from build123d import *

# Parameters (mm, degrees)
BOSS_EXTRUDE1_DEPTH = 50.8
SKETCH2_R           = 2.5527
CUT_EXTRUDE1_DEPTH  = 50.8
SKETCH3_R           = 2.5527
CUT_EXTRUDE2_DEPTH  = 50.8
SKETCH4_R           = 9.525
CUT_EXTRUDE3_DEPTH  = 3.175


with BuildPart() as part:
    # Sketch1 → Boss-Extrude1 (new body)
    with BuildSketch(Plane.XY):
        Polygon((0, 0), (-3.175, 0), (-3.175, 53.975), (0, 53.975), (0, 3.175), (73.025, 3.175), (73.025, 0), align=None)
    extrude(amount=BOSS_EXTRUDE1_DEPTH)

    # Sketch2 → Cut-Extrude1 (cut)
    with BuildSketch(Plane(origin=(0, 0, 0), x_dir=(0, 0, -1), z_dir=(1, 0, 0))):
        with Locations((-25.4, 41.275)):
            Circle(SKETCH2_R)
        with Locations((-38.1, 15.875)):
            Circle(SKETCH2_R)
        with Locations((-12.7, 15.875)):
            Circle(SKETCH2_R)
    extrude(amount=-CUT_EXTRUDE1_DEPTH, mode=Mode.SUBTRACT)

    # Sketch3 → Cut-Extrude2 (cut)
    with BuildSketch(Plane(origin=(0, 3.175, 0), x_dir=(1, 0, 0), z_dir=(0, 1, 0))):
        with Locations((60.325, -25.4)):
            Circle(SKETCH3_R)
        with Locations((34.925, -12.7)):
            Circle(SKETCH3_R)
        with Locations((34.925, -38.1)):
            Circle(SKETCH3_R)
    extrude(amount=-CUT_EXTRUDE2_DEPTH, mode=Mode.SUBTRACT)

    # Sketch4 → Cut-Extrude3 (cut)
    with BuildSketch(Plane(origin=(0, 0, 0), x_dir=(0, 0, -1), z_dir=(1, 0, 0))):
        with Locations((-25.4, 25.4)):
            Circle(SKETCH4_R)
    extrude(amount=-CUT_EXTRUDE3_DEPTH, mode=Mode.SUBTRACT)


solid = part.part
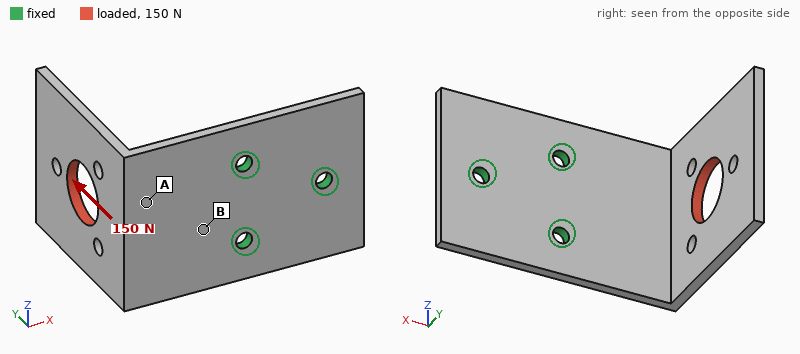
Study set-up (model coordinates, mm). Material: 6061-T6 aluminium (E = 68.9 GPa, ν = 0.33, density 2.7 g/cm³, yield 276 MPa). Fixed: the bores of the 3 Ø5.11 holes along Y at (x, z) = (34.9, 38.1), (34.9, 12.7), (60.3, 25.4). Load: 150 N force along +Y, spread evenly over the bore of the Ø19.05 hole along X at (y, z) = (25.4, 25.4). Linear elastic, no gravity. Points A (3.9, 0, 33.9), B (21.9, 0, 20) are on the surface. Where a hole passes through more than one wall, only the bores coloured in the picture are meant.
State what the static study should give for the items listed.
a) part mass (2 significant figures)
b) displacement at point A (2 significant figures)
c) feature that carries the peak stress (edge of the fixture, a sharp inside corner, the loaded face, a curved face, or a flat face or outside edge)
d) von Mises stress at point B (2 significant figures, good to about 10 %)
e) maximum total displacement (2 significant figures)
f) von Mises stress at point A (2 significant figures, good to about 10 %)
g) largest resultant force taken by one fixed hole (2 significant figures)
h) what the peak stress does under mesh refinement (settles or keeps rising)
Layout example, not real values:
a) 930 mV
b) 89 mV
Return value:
a) 52 g
b) 0.19 mm
c) edge of the fixture
d) 37 MPa
e) 0.57 mm
f) 9.1 MPa
g) 88 N
h) keeps rising
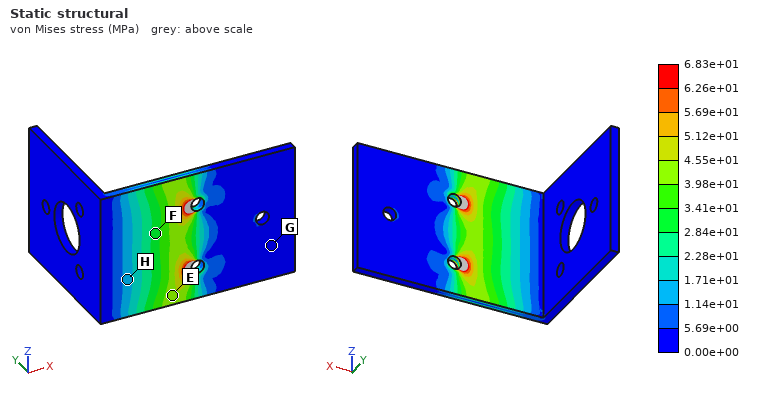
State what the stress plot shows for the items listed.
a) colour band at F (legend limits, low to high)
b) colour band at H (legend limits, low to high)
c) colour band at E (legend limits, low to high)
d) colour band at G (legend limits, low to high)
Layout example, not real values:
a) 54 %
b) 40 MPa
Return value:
a) 2.84e+01 to 3.41e+01 MPa
b) 1.14e+01 to 1.71e+01 MPa
c) 3.98e+01 to 4.55e+01 MPa
d) 0.00e+00 to 5.69e+00 MPa
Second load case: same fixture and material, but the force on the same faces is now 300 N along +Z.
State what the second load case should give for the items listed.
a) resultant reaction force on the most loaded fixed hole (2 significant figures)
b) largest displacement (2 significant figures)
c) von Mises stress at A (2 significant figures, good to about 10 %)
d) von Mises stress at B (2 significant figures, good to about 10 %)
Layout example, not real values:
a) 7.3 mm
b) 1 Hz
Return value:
a) 420 N
b) 0.62 mm
c) 41 MPa
d) 43 MPa
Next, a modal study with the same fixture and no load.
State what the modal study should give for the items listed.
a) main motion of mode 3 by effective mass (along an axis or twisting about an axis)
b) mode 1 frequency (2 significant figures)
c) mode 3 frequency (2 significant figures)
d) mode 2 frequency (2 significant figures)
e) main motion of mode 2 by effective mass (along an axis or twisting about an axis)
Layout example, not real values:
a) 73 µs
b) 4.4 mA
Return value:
a) along Y
b) 460 Hz
c) 1300 Hz
d) 820 Hz
e) along Z
